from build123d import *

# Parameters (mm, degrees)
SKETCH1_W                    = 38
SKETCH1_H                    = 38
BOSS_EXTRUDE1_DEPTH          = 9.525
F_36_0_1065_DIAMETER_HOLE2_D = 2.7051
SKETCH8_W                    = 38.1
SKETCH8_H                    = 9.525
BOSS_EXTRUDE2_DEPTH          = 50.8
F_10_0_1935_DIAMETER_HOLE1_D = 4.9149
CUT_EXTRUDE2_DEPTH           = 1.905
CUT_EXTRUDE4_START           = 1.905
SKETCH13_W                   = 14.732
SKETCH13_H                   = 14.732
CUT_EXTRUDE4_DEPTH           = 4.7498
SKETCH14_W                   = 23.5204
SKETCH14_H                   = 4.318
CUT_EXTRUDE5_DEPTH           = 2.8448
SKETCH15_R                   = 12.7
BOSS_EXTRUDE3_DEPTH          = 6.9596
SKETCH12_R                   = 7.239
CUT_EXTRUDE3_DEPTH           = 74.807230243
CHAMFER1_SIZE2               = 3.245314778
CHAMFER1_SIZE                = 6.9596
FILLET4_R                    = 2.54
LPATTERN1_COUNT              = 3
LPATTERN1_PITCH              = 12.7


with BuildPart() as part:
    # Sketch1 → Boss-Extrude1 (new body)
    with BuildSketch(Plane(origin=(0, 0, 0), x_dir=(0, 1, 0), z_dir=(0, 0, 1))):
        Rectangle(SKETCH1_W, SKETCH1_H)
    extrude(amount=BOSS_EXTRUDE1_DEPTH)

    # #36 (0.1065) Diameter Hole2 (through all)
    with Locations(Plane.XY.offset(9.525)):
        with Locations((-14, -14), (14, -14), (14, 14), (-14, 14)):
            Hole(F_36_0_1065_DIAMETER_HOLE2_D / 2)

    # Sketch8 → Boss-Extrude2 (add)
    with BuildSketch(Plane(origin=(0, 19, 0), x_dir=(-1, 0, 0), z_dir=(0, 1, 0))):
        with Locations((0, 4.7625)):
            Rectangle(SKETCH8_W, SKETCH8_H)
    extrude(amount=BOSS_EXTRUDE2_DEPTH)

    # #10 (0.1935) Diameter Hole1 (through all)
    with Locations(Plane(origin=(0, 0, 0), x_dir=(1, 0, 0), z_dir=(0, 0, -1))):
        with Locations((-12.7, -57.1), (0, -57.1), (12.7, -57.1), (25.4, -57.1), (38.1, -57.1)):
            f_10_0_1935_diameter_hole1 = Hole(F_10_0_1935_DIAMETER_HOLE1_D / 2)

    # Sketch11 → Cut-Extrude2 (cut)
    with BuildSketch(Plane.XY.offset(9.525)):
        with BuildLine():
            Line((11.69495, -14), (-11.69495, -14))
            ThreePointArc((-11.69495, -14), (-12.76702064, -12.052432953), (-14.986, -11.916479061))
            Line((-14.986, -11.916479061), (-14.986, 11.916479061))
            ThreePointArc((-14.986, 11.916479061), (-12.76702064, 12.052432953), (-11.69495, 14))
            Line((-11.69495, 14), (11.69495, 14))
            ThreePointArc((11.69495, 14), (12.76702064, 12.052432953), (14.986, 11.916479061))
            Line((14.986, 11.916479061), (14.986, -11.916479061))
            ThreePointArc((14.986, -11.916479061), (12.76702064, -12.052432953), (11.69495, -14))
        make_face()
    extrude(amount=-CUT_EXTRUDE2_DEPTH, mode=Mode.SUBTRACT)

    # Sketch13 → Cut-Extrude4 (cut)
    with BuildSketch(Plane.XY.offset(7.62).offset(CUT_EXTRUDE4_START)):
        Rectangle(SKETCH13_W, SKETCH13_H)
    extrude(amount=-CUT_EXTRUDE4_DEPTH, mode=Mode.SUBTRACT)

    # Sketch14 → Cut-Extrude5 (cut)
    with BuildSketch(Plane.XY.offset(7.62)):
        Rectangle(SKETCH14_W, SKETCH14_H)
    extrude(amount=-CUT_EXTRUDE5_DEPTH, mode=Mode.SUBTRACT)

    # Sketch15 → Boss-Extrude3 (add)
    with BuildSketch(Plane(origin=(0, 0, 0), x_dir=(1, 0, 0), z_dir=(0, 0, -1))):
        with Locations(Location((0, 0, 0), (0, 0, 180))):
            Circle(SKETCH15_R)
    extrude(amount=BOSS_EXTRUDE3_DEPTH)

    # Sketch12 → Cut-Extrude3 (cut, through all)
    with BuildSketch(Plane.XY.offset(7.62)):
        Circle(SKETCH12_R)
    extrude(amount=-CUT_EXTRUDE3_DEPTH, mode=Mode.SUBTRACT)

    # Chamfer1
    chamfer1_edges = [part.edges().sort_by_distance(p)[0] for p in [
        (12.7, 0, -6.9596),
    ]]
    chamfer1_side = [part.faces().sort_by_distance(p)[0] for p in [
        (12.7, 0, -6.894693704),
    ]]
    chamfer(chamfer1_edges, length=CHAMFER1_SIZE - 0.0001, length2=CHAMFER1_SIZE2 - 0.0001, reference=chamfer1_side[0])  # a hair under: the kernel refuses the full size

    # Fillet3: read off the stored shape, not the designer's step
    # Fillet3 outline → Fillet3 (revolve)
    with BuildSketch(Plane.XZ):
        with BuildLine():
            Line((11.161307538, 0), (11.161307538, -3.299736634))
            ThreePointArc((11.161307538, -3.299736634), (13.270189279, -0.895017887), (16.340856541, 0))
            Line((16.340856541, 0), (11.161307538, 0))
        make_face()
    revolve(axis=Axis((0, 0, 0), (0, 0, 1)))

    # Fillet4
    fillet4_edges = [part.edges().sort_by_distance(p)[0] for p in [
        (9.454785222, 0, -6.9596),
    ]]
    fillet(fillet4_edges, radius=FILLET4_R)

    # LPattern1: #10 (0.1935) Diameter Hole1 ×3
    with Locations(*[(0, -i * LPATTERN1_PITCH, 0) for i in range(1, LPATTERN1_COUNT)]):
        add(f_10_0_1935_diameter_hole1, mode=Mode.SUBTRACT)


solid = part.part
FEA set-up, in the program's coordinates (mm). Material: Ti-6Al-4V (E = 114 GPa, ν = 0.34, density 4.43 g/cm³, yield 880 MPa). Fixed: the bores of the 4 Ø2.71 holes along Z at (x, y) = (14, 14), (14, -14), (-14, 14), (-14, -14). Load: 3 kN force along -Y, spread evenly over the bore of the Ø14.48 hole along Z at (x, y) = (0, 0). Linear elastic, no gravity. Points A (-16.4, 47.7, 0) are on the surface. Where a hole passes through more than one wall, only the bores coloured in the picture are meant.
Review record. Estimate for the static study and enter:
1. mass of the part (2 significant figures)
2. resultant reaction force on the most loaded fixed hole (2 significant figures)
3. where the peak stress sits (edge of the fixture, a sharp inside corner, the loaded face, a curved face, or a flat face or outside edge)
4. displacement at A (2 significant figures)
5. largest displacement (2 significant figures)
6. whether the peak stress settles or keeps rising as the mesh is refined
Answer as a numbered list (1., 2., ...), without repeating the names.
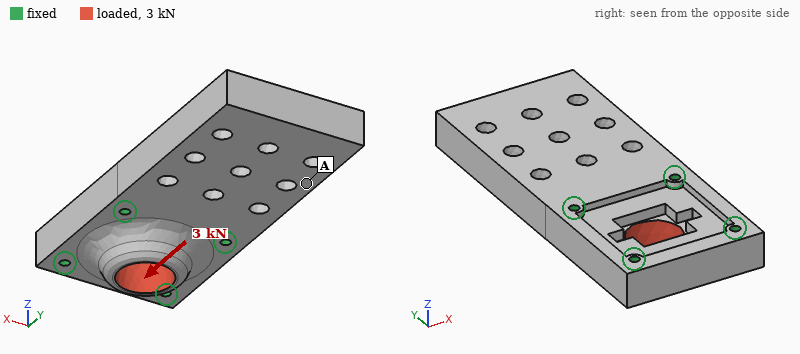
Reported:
1. 130 g
2. 860 N
3. edge of the fixture
4. 1.7 µm
5. 3.9 µm
6. keeps rising
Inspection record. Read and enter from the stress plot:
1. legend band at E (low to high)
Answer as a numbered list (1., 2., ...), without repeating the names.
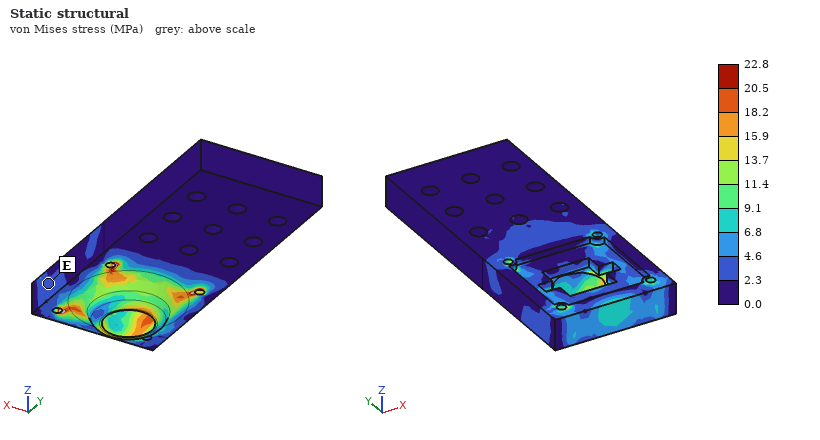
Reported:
1. 2.3 to 4.6 MPa
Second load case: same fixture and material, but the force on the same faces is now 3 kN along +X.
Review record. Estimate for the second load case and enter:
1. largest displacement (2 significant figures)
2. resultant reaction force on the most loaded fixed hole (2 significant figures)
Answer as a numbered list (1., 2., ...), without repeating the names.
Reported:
1. 3.9 µm
2. 850 N
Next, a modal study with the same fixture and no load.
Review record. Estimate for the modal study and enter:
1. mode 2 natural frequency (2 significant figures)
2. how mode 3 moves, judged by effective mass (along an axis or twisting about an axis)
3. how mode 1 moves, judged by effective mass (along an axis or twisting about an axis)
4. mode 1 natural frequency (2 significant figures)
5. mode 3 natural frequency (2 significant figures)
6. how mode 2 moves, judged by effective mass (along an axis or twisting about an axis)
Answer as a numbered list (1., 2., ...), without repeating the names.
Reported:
1. 6600 Hz
2. along X
3. along Z
4. 2200 Hz
5. 7100 Hz
6. twisting about Y
